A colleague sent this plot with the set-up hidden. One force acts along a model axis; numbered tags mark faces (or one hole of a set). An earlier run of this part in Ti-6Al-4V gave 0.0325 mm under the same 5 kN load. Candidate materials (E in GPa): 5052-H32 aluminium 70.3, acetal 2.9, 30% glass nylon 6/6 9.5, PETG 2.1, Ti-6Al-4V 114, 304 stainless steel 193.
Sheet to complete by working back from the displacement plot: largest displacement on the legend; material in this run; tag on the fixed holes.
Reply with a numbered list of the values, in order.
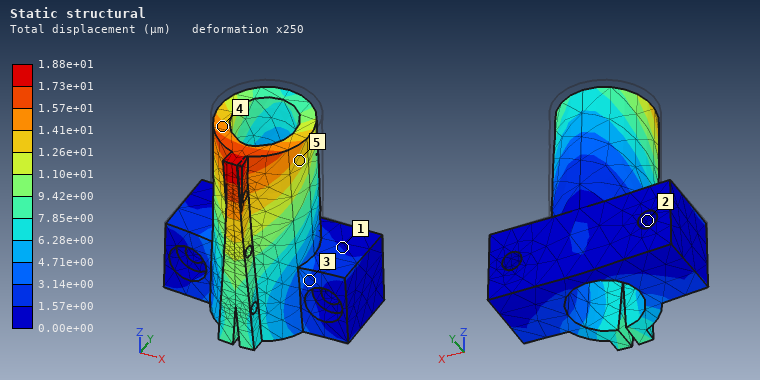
1. 1.88e+01 µm
2. 304 stainless steel
3. 2
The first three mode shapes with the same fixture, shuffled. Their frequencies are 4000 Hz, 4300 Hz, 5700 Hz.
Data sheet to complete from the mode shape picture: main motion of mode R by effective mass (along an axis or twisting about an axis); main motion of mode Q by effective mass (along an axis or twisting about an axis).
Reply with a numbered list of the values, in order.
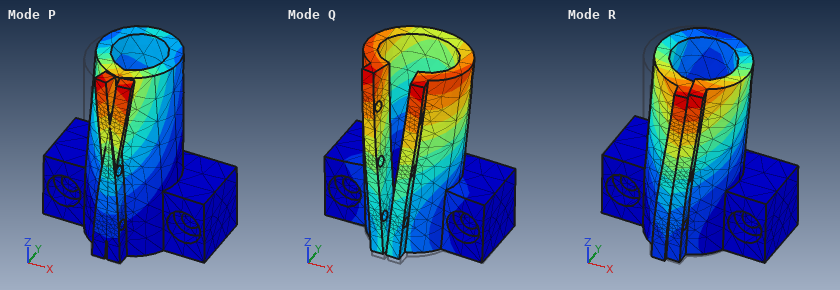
1. along X
2. along Y
